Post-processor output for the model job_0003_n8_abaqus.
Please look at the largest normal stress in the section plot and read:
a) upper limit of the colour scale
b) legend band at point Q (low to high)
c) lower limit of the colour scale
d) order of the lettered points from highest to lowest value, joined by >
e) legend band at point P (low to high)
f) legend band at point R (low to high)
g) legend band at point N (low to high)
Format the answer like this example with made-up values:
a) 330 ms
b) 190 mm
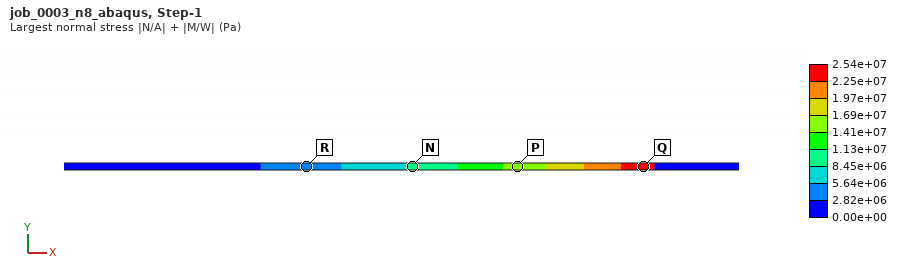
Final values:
a) 2.54e+07 Pa
b) 2.25e+07 to 2.54e+07 Pa
c) 0.00e+00 Pa
d) Q > P > N > R
e) 1.41e+07 to 1.69e+07 Pa
f) 2.82e+06 to 5.64e+06 Pa
g) 8.45e+06 to 1.13e+07 Pa
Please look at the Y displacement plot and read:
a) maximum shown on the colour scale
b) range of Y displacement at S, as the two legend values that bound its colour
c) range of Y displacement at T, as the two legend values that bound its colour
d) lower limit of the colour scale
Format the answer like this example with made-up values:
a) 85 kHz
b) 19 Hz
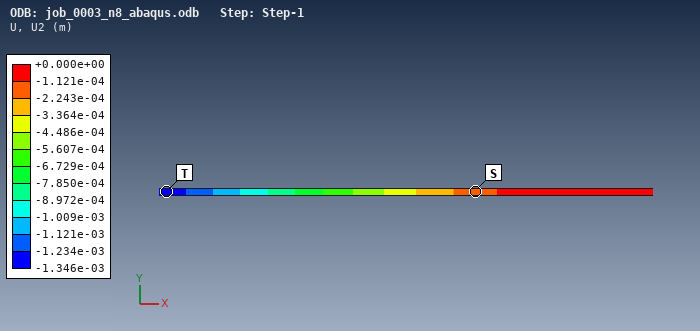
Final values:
a) +0.000e+00 m
b) -2.243e-04 to -1.121e-04 m
c) -1.346e-03 to -1.234e-03 m
d) -1.346e-03 m
